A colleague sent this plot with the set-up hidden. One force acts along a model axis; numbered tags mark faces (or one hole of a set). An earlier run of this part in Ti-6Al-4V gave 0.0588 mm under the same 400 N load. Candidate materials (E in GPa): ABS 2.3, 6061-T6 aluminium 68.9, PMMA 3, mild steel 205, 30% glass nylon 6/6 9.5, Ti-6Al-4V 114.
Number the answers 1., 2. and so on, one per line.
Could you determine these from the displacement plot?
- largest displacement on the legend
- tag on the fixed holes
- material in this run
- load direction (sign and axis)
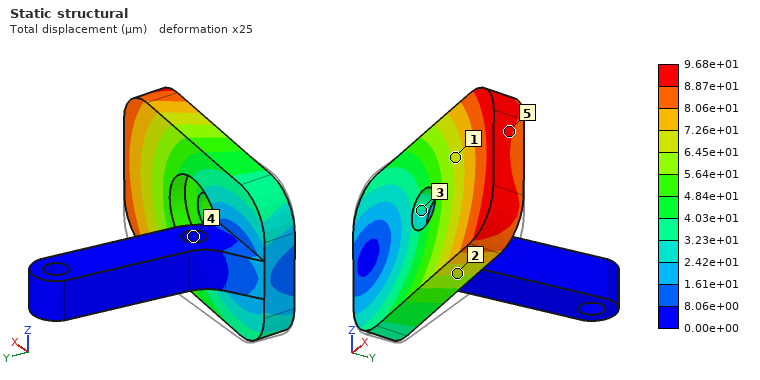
1. 9.68e+01 µm
2. 4
3. 6061-T6 aluminium
4. +Z
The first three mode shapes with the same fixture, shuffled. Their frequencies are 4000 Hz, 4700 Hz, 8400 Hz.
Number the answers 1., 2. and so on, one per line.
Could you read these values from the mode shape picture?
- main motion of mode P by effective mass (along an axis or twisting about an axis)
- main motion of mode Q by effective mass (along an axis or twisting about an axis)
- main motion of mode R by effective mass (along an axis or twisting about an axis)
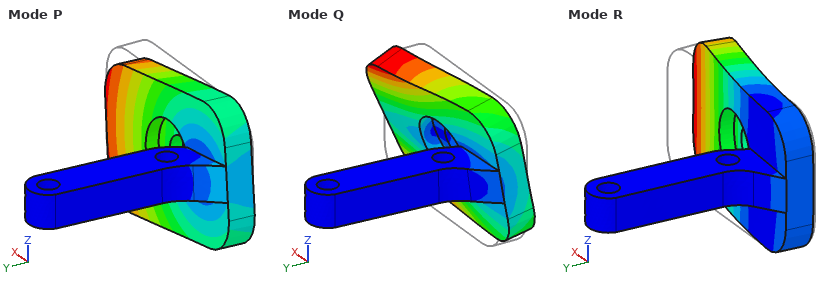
1. along Z
2. twisting about X
3. along Y
